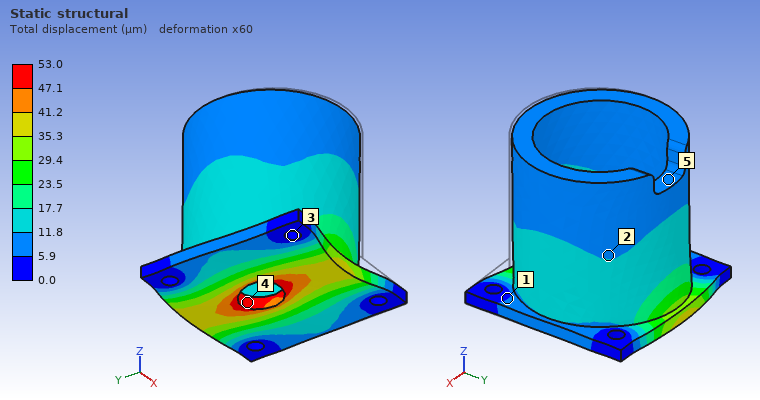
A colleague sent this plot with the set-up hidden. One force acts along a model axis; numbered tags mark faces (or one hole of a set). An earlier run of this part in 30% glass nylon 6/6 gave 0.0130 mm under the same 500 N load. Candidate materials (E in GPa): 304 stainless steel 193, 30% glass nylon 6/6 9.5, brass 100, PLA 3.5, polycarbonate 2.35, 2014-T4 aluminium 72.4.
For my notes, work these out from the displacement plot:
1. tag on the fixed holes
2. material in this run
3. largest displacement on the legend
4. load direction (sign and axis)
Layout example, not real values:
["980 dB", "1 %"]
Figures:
["3", "polycarbonate", "53.0 µm", "+Y"]
